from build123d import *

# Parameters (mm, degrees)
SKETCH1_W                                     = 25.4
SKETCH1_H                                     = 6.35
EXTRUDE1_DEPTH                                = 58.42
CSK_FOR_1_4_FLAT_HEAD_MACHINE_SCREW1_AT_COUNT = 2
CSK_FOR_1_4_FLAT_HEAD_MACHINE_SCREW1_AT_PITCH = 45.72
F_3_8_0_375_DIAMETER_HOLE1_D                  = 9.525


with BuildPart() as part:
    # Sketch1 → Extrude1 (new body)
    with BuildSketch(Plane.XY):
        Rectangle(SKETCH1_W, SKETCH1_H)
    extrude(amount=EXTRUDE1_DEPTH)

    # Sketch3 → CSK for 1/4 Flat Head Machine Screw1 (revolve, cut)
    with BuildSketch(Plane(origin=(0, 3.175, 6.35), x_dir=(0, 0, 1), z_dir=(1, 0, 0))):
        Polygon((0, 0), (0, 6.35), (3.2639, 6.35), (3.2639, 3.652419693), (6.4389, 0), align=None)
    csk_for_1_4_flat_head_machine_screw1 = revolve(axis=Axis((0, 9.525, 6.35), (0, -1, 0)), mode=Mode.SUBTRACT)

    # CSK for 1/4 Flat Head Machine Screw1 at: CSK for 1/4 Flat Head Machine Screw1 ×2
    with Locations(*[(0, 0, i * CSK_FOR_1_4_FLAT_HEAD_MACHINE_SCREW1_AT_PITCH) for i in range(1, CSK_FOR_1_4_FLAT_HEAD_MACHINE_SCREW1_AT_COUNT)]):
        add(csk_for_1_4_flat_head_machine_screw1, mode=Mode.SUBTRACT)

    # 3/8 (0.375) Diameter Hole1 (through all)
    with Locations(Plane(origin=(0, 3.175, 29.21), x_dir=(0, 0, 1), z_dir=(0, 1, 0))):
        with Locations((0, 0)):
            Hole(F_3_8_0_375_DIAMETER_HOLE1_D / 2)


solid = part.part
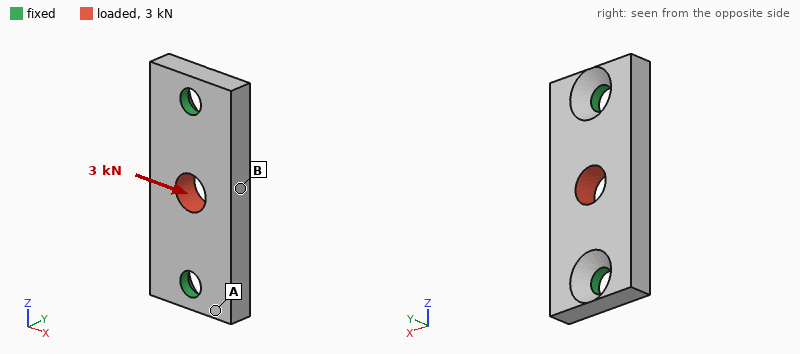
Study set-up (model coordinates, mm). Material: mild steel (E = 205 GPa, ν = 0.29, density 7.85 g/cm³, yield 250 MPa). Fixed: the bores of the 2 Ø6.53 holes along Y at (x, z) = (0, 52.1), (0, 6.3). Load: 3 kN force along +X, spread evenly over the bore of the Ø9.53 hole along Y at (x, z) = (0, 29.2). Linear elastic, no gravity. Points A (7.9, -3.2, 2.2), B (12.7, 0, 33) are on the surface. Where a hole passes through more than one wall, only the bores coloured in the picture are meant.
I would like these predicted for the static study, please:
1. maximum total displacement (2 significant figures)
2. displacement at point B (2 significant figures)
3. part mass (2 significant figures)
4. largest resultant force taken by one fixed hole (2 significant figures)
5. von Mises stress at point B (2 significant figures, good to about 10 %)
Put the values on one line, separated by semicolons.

7.3 µm; 6.2 µm; 65 g; 1.5 kN; 38 MPa
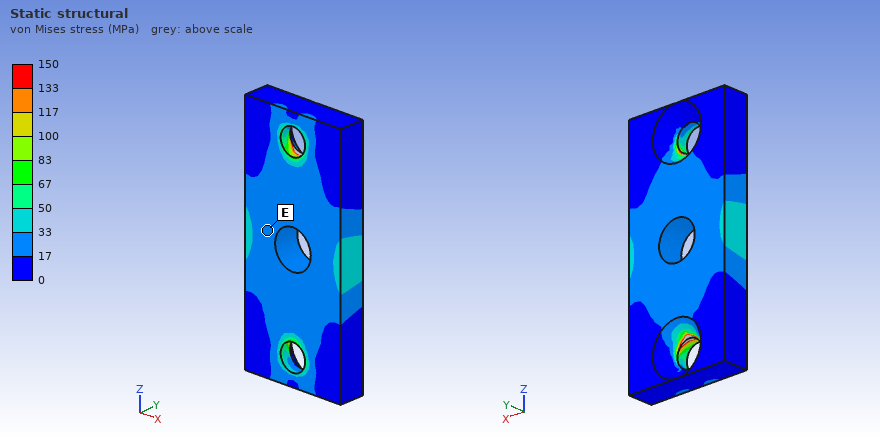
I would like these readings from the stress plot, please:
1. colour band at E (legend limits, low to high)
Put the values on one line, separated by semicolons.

17 to 33 MPa
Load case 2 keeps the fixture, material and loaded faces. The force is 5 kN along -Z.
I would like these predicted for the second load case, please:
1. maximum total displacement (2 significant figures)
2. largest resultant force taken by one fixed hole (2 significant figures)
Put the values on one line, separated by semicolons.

3.3 µm; 2.5 kN
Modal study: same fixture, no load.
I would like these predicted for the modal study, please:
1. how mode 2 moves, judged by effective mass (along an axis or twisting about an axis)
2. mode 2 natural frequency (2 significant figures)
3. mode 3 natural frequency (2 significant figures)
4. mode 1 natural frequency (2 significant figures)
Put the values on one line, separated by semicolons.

along Y; 11 kHz; 20 kHz; 11 kHz
